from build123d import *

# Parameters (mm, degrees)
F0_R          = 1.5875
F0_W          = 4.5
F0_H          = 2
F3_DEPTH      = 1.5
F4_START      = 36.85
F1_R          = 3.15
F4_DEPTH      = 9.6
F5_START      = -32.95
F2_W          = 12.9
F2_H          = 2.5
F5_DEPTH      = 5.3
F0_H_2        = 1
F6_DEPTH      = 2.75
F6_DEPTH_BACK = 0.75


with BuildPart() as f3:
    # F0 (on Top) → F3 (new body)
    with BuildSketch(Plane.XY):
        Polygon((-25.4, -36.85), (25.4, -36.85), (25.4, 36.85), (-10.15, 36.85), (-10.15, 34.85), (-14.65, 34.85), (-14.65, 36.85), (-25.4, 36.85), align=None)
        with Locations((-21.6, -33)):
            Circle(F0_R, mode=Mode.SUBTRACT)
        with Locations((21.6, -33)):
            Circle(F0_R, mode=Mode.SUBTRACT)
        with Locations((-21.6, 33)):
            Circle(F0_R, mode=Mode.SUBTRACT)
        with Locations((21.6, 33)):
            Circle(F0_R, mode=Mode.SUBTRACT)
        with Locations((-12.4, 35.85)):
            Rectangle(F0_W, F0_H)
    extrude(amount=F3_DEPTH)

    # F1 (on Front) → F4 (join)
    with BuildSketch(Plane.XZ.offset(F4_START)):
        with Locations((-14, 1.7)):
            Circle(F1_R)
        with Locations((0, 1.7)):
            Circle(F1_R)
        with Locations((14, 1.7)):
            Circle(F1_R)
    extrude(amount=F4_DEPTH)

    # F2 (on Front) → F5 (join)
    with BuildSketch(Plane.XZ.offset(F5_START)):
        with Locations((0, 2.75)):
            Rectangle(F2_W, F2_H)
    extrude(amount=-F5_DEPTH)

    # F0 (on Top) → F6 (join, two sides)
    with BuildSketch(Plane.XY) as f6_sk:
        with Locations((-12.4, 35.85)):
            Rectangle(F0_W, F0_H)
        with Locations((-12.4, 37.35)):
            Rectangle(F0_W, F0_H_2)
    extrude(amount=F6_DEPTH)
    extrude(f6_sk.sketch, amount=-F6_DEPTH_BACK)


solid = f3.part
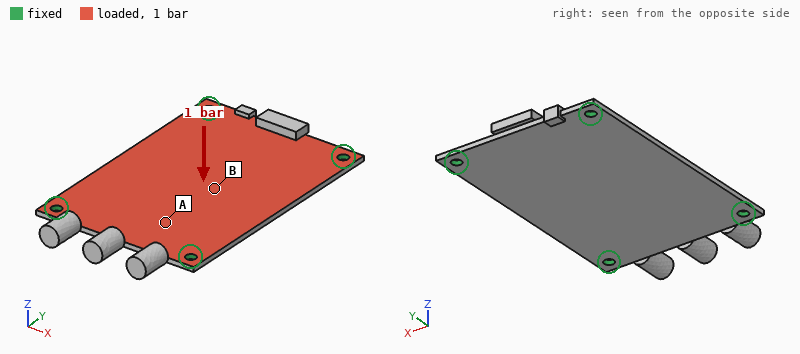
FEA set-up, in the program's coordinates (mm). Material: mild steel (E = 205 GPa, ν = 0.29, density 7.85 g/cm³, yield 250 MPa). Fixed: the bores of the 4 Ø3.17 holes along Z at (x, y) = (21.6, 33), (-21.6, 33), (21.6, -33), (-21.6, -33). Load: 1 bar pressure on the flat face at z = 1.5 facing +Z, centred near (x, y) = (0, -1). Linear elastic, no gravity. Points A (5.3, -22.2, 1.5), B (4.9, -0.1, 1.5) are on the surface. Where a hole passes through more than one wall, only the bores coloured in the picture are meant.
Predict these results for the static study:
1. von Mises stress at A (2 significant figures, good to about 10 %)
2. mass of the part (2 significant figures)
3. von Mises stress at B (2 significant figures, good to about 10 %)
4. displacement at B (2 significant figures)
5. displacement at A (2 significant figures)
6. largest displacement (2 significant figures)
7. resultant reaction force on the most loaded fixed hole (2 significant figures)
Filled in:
25 MPa
52 g
49 MPa
0.12 mm
0.061 mm
0.12 mm
93 N
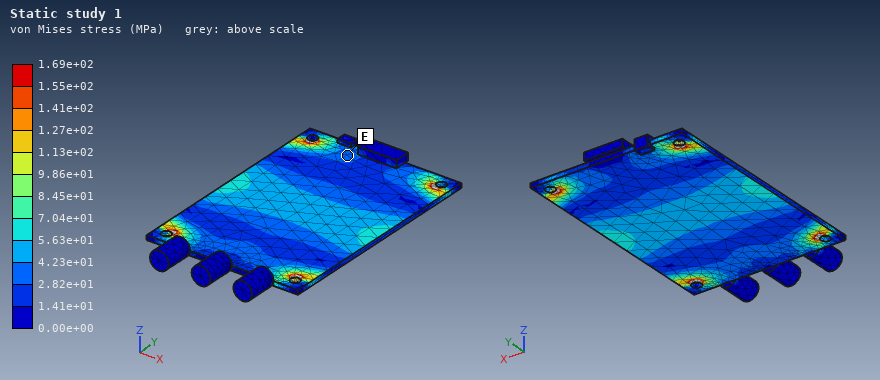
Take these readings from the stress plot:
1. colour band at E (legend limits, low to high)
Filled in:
2.82e+01 to 4.23e+01 MPa
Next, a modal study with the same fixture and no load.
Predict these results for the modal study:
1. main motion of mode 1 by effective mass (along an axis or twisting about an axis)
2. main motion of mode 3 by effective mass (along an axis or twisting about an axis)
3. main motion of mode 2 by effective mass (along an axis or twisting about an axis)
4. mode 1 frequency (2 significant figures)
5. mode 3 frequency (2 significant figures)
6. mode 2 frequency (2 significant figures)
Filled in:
along Z
twisting about Y
along Z
1500 Hz
2500 Hz
2400 Hz
